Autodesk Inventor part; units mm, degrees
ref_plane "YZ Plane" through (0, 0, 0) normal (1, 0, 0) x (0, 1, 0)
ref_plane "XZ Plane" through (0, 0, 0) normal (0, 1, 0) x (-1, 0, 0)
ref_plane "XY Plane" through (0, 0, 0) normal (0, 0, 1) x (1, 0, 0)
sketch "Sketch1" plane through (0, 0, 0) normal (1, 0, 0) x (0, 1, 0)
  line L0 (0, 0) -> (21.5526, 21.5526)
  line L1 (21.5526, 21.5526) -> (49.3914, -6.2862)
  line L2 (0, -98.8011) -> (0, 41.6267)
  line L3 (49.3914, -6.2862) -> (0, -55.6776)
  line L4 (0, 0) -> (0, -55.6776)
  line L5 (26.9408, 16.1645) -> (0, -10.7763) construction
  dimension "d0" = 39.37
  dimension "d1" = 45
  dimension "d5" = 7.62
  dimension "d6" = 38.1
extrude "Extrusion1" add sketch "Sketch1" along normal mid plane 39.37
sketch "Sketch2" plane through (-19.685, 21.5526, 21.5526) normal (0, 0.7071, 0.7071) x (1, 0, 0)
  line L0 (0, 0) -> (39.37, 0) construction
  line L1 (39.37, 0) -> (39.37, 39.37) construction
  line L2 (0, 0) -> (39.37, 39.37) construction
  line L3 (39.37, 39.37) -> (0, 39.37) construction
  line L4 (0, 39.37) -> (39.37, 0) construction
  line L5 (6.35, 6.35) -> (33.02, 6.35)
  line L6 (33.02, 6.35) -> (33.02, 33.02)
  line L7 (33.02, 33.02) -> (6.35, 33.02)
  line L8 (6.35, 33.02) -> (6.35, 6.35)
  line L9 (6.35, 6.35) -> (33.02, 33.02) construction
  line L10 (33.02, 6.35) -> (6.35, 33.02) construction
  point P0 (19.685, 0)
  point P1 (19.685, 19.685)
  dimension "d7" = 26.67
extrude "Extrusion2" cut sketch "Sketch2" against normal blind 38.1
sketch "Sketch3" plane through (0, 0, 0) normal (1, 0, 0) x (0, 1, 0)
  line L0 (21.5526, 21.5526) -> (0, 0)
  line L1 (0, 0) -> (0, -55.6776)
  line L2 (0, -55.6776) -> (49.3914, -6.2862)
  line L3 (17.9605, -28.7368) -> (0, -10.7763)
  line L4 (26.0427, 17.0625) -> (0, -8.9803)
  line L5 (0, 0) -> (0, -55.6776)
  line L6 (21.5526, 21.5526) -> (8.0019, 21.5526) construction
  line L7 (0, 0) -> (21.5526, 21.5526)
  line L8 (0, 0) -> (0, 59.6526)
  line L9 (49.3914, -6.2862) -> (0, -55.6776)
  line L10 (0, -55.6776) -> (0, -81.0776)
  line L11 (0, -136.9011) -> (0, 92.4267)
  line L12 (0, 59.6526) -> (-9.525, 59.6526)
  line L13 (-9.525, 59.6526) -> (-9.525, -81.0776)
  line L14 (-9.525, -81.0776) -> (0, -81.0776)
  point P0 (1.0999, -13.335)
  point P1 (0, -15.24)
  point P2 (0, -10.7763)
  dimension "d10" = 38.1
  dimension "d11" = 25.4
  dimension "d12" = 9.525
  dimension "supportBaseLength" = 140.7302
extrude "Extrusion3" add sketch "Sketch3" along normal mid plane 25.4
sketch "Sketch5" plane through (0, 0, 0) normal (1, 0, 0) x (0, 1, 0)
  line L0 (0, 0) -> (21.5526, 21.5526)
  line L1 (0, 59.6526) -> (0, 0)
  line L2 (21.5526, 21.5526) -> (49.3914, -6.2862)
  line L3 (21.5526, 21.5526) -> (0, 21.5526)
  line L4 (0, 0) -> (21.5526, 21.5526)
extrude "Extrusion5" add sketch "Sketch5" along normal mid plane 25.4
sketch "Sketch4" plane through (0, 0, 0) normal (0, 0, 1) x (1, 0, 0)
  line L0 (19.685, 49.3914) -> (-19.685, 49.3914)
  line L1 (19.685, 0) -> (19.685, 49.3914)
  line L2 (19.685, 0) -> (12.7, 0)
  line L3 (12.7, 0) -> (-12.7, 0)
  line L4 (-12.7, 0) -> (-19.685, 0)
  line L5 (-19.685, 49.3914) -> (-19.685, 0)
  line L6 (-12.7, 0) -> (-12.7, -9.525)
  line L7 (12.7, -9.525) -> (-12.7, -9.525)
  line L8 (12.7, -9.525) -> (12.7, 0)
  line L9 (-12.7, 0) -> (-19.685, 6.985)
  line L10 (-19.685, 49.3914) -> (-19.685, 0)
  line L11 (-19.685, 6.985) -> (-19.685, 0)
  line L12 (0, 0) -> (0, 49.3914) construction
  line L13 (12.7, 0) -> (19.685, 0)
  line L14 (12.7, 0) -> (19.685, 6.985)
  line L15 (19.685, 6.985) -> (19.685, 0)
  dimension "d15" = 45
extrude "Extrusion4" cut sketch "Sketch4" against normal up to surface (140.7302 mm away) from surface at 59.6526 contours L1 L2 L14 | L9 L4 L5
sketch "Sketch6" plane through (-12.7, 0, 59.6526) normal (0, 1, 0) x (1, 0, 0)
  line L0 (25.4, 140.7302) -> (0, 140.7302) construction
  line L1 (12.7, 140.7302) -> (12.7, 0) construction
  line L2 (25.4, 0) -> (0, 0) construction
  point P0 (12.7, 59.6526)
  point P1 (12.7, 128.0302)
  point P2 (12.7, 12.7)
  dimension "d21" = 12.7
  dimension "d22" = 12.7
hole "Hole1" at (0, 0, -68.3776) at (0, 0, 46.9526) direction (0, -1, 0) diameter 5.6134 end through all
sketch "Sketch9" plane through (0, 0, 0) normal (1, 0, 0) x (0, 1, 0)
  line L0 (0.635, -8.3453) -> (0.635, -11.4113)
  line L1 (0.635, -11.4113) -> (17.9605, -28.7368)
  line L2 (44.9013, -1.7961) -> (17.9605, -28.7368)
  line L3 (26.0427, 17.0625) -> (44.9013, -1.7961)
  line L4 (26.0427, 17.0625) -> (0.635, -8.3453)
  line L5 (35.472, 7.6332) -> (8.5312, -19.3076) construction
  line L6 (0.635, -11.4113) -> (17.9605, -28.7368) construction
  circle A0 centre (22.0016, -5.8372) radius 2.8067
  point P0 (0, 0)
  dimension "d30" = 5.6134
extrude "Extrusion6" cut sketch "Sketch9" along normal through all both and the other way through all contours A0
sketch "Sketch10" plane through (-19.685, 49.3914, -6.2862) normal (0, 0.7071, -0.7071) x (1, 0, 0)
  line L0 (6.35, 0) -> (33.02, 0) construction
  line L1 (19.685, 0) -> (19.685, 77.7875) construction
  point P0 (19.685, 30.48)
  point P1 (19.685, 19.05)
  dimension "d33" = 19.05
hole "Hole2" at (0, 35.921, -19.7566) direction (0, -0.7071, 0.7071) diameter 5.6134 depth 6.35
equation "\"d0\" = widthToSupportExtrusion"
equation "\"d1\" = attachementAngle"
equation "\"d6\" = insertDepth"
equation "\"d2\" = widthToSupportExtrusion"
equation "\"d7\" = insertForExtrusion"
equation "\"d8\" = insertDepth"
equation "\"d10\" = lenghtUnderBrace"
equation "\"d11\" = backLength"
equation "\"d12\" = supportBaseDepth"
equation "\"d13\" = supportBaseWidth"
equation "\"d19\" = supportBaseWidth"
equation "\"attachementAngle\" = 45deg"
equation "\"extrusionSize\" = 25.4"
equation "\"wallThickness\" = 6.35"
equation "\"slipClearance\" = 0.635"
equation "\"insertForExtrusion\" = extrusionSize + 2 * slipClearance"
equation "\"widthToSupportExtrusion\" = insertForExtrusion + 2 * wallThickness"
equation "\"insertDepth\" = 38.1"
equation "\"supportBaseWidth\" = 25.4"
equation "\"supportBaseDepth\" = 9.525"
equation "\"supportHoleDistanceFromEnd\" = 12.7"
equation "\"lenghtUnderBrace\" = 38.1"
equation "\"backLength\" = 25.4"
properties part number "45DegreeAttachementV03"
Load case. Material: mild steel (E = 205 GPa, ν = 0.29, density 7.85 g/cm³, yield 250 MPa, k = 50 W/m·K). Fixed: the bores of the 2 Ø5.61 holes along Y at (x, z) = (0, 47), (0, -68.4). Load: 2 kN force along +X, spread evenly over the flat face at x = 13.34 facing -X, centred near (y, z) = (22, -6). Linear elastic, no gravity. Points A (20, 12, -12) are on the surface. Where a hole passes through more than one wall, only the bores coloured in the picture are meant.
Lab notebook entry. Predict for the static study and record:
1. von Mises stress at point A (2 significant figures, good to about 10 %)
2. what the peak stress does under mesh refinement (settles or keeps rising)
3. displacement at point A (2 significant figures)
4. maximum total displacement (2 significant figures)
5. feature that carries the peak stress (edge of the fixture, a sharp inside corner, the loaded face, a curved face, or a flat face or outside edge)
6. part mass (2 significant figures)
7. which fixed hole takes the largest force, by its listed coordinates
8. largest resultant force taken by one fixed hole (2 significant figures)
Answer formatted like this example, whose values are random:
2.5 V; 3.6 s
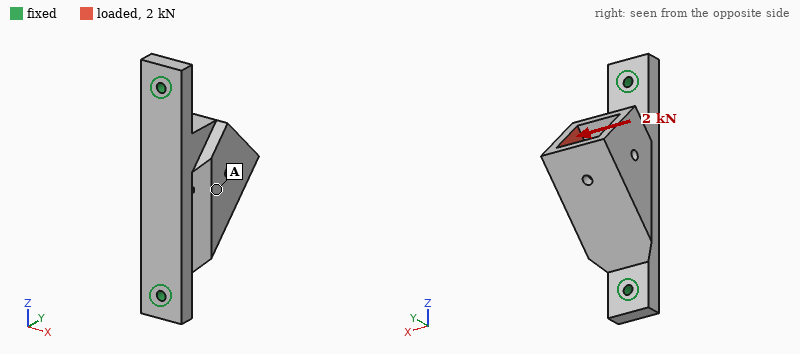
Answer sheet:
16 MPa; keeps rising; 39 µm; 81 µm; edge of the fixture; 680 g; (0, 47); 1.1 kN
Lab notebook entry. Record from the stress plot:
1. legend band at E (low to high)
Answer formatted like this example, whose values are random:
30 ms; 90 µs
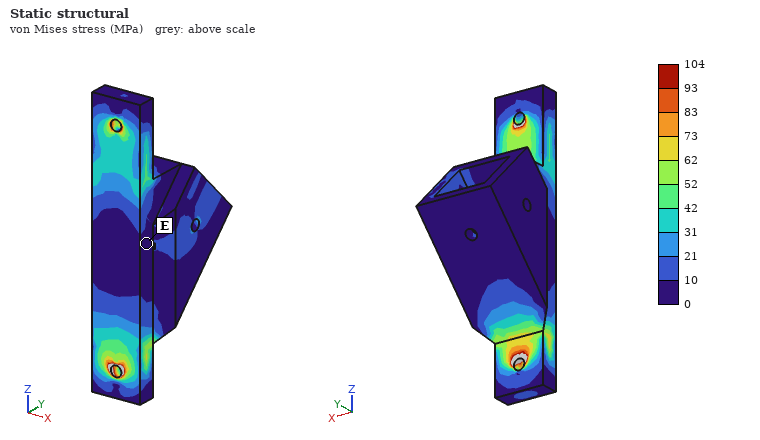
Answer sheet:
0 to 10 MPa
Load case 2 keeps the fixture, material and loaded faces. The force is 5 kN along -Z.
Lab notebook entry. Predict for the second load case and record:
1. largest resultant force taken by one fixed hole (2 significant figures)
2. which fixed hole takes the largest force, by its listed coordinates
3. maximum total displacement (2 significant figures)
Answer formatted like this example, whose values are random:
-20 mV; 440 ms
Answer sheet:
3.2 kN; (0, -68.4); 17 µm
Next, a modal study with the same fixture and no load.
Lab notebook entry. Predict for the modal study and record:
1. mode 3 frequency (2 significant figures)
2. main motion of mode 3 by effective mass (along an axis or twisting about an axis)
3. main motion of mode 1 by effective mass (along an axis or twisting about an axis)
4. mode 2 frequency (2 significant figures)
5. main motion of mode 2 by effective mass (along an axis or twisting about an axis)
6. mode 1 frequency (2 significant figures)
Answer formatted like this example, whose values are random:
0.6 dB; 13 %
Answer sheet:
5600 Hz; along X; along X; 3500 Hz; along Y; 1700 Hz
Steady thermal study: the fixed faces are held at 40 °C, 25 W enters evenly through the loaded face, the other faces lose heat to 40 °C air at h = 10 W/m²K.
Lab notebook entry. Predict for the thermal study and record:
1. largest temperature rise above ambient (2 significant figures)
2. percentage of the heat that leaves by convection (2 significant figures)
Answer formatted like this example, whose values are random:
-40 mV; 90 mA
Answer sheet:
48 K; 20 %
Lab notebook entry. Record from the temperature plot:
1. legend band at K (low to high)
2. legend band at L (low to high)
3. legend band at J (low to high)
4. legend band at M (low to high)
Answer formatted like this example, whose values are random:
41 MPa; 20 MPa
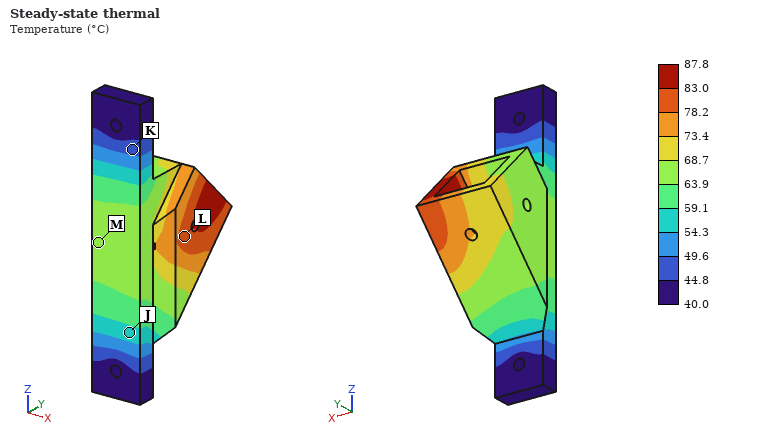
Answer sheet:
44.8 to 49.6 °C; 78.2 to 83.0 °C; 54.3 to 59.1 °C; 63.9 to 68.7 °C
